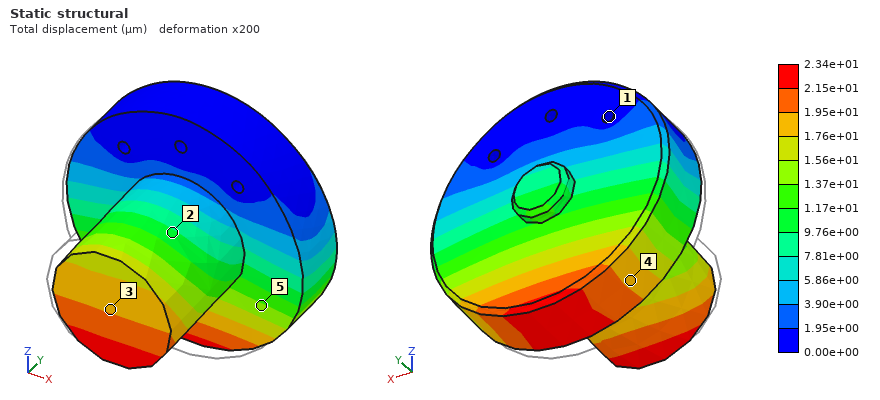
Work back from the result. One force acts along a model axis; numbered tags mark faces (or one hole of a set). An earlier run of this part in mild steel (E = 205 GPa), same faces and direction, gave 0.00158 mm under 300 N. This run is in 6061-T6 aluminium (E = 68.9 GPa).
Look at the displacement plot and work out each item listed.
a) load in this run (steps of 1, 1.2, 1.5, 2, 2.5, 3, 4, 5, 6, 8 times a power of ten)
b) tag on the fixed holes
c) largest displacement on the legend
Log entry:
1.5 kN
1
2.34e+01 µm
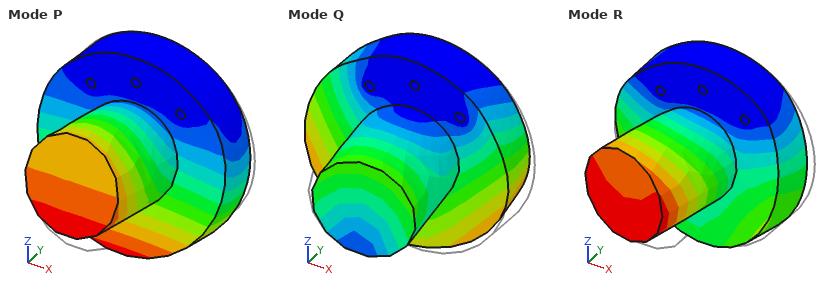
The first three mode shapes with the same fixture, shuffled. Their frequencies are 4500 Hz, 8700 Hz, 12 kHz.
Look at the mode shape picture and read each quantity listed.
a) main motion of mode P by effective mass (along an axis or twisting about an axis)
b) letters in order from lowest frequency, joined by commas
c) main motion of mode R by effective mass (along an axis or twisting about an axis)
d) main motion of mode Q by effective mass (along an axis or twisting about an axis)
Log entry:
along Y
P, R, Q
along X
along X
